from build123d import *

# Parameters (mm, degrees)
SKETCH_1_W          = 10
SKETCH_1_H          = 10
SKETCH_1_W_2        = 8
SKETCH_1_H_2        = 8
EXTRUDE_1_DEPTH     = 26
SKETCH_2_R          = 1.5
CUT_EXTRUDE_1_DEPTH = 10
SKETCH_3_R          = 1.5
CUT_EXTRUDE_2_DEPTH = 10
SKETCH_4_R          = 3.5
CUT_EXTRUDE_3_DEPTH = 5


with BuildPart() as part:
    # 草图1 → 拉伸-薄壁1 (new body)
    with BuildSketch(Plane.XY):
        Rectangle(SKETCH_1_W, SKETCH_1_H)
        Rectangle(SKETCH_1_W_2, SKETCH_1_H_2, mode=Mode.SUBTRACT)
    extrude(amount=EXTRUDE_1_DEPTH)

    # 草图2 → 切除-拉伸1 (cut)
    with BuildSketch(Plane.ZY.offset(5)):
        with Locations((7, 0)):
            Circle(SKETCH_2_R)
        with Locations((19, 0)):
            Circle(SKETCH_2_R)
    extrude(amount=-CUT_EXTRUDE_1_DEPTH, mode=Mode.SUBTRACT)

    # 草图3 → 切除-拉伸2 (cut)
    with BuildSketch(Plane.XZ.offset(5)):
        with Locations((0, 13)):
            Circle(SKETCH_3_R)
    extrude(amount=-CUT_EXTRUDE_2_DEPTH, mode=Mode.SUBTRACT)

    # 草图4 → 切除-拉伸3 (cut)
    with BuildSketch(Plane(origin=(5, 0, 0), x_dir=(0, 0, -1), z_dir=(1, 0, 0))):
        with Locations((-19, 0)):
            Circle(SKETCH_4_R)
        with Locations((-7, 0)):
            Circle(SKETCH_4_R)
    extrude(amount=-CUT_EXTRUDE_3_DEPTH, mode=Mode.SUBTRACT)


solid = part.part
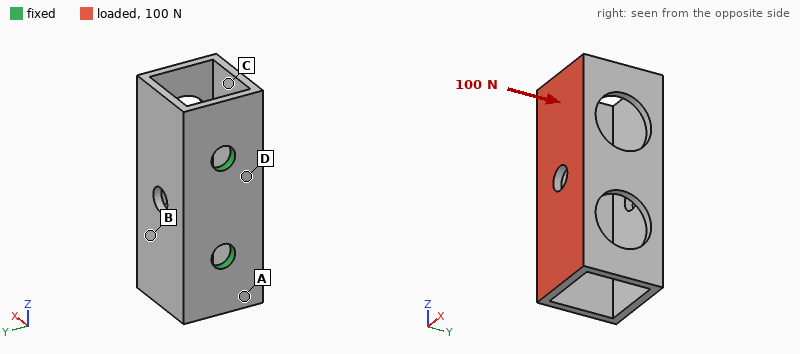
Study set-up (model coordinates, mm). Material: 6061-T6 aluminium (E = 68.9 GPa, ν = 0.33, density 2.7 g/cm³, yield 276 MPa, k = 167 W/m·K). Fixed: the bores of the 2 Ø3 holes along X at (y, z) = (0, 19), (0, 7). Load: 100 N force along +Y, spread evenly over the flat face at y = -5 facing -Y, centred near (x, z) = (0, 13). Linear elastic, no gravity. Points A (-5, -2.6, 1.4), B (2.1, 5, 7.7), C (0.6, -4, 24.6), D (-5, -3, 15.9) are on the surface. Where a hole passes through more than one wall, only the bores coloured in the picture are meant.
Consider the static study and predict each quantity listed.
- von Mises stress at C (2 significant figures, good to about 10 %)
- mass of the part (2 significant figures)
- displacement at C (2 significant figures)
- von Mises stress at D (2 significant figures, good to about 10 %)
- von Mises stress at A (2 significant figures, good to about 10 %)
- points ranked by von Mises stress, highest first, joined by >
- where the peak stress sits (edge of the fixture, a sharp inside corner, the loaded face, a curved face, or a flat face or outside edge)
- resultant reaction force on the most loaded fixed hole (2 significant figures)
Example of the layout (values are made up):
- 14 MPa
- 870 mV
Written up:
- 17 MPa
- 2.2 g
- 30 µm
- 37 MPa
- 27 MPa
- D > A > C > B
- a flat face or outside edge
- 50 N
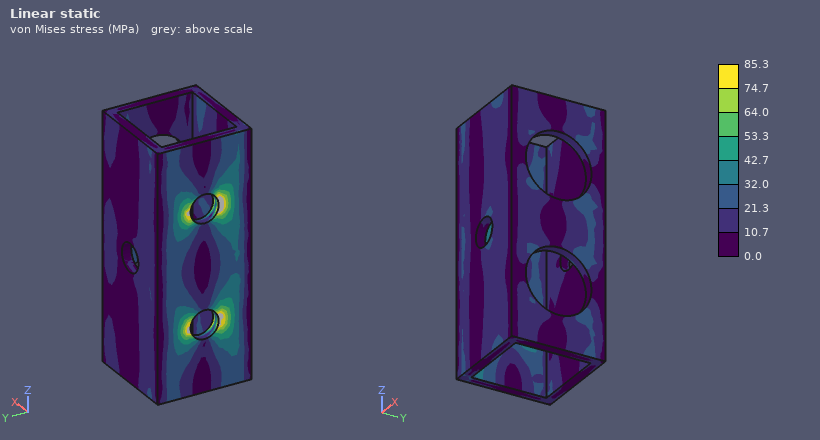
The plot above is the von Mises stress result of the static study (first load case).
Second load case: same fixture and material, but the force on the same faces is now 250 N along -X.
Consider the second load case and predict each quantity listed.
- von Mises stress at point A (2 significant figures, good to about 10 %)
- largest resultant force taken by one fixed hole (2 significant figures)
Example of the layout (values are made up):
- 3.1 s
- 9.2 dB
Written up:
- 36 MPa
- 130 N
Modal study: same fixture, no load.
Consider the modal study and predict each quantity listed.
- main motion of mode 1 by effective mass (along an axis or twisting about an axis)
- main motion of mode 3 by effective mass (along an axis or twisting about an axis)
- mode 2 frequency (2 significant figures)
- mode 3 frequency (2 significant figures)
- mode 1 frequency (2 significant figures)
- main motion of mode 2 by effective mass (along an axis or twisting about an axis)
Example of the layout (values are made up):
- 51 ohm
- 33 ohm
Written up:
- along Y
- twisting about X
- 12 kHz
- 15 kHz
- 5600 Hz
- along Z
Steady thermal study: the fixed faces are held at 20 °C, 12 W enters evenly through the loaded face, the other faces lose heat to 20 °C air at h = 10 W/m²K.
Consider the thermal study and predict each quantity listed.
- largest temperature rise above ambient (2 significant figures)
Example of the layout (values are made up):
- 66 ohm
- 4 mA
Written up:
- 19 K
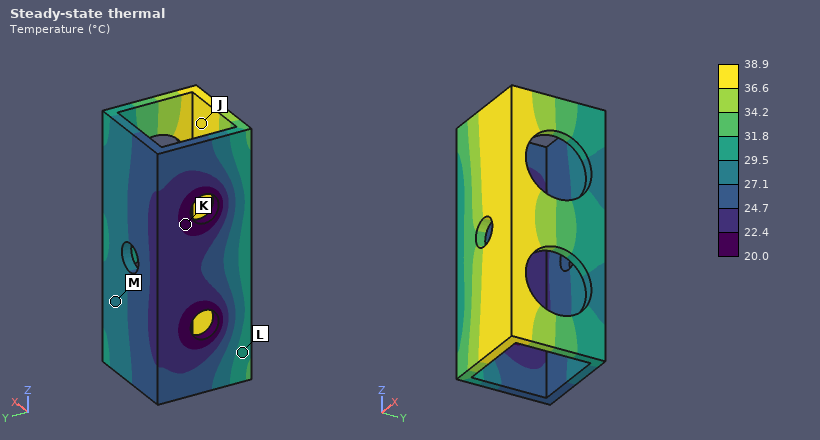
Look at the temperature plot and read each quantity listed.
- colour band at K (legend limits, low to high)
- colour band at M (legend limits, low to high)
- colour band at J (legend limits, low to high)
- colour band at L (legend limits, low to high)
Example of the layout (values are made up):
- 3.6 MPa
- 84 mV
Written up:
- 20.0 to 22.4 °C
- 27.1 to 29.5 °C
- 36.6 to 38.9 °C
- 29.5 to 31.8 °C
